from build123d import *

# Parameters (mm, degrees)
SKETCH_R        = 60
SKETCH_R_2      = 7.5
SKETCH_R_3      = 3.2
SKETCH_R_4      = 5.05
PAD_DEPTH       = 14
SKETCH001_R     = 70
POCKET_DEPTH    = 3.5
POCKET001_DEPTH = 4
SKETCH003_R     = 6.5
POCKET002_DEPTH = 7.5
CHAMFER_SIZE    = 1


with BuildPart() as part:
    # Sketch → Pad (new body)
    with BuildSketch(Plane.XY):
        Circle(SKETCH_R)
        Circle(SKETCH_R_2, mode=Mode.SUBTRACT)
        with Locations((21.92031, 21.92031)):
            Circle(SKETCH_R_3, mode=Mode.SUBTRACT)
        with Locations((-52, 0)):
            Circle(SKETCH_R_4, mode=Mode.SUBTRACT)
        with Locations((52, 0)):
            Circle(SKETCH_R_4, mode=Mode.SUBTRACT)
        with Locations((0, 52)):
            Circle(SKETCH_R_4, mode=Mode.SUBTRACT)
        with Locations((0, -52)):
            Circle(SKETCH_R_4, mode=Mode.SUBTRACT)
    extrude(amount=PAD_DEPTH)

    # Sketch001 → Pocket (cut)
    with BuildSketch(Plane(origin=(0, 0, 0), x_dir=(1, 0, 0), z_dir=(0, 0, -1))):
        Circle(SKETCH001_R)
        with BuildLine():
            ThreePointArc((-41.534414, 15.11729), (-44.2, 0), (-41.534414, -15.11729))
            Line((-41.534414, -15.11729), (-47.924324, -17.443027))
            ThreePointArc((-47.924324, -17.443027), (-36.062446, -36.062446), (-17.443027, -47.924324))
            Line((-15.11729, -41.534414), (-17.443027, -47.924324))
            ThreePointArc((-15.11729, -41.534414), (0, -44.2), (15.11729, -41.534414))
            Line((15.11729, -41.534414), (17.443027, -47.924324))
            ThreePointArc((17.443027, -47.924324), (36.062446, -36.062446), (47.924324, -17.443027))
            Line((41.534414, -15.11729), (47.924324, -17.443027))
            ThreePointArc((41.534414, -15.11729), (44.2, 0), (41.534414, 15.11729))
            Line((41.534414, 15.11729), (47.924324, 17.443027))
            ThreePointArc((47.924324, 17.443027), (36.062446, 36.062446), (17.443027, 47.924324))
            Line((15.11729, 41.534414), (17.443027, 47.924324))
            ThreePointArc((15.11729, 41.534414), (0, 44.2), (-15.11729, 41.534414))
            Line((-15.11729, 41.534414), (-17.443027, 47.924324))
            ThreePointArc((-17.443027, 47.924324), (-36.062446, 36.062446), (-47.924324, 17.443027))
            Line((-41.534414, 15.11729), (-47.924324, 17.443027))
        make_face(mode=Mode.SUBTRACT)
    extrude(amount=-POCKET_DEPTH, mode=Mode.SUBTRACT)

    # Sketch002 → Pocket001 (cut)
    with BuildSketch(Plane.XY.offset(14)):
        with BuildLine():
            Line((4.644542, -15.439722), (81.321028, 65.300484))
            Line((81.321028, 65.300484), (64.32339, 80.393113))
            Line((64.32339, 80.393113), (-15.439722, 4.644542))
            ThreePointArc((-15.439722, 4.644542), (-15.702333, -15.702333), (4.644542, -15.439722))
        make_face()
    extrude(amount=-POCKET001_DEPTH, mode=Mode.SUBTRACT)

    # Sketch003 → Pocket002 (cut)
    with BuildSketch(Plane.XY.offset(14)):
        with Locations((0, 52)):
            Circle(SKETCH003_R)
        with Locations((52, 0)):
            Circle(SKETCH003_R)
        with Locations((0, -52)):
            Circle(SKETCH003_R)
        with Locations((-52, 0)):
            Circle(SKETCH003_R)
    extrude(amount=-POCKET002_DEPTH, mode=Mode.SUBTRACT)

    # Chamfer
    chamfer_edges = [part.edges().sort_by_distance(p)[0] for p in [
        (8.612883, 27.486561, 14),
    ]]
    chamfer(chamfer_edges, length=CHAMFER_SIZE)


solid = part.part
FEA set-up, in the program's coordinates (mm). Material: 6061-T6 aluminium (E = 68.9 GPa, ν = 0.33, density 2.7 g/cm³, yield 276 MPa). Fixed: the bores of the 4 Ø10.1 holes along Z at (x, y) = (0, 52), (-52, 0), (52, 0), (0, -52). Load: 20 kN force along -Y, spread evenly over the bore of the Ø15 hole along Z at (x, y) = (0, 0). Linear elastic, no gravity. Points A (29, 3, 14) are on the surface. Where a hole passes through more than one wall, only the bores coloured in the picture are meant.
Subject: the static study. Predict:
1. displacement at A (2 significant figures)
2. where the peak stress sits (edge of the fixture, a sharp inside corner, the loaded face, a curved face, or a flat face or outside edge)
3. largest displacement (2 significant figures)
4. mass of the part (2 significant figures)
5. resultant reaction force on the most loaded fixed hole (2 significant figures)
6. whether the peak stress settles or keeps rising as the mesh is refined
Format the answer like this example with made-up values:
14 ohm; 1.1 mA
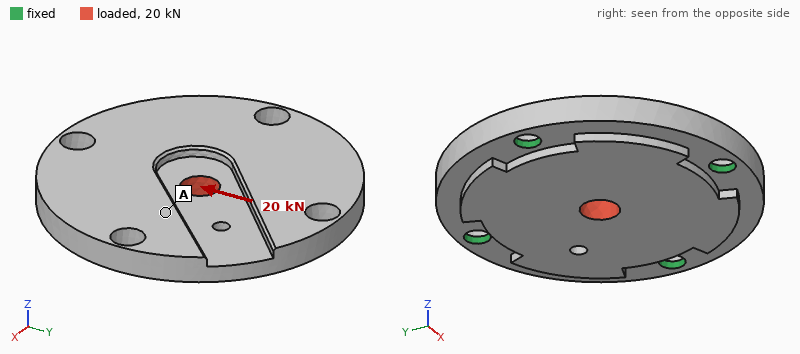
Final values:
9.5 µm; edge of the fixture; 23 µm; 350 g; 6.2 kN; keeps rising
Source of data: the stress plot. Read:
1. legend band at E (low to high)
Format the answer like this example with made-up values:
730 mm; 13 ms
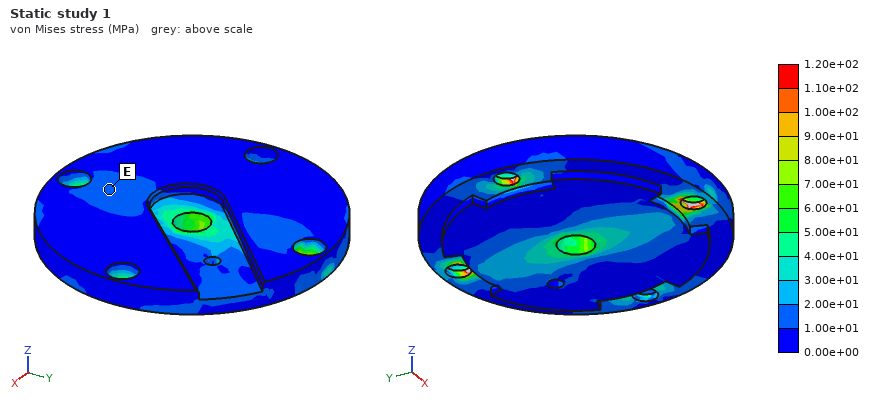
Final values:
1.00e+01 to 2.00e+01 MPa
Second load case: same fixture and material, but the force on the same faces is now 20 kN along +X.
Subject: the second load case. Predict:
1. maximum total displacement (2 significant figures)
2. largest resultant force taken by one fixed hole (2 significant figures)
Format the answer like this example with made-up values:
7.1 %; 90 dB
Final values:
23 µm; 6.2 kN
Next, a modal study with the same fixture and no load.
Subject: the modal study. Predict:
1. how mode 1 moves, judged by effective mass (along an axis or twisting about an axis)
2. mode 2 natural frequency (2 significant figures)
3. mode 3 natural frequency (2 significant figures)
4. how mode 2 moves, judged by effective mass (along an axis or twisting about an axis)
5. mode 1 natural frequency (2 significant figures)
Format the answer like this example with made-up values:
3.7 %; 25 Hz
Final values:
along Z; 6100 Hz; 7000 Hz; along Z; 5300 Hz
